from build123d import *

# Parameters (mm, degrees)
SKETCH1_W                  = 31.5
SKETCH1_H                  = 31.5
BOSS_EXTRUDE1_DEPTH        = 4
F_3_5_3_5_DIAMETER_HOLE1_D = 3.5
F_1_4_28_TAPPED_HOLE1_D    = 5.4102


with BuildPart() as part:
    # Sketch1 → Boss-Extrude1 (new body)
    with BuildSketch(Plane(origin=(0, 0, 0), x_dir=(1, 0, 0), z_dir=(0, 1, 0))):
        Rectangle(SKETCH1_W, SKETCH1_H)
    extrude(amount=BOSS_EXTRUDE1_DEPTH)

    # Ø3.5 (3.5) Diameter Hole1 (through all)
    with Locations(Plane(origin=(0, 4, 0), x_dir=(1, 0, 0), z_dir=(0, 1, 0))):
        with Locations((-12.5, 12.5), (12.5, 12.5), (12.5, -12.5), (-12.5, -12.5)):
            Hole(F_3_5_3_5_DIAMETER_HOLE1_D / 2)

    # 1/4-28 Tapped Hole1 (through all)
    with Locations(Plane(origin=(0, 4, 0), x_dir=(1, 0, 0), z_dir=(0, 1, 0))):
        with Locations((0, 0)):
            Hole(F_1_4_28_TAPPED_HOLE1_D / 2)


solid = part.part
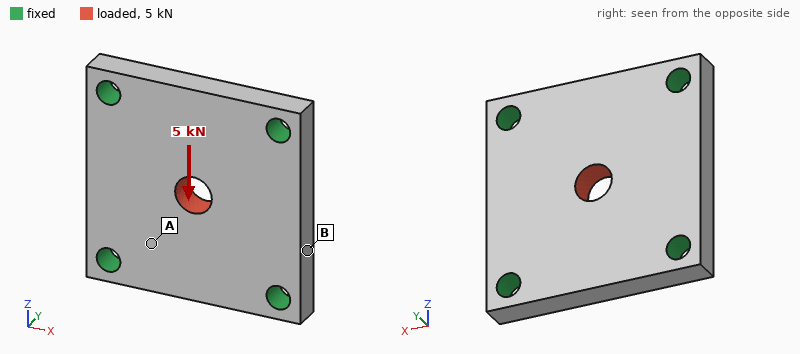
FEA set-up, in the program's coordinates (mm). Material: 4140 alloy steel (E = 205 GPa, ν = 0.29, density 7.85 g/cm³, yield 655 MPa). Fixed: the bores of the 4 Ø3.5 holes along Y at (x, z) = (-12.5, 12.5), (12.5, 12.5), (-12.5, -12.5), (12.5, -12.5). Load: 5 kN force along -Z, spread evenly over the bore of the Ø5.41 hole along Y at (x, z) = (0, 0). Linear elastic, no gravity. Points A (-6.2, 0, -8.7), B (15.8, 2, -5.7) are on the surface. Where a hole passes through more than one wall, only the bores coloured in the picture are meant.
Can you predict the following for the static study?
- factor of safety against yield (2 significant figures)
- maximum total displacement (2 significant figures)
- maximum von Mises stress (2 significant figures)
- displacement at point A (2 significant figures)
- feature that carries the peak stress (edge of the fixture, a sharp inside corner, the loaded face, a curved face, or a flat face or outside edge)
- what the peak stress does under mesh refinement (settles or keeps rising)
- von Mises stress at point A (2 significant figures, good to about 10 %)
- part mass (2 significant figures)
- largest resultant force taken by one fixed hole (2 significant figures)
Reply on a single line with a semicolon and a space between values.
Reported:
5.1; 4.4 µm; 130 MPa; 2.0 µm; the loaded face; settles; 43 MPa; 29 g; 1.4 kN
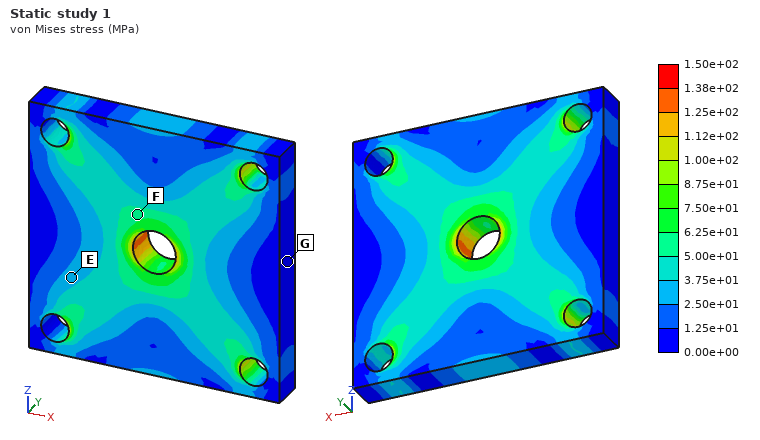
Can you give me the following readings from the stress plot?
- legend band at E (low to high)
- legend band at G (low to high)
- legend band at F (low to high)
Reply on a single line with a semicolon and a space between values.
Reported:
2.50e+01 to 3.75e+01 MPa; 0.00e+00 to 1.25e+01 MPa; 5.00e+01 to 6.25e+01 MPa
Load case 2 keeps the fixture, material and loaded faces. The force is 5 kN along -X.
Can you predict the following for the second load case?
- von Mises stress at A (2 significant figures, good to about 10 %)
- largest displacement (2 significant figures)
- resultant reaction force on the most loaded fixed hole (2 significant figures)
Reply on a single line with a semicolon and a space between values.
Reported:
41 MPa; 4.4 µm; 1.4 kN
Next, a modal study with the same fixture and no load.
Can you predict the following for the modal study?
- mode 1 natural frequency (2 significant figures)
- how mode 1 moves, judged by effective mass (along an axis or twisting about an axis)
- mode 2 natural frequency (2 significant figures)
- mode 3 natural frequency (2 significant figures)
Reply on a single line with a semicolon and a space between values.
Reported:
22 kHz; along Y; 35 kHz; 35 kHz
